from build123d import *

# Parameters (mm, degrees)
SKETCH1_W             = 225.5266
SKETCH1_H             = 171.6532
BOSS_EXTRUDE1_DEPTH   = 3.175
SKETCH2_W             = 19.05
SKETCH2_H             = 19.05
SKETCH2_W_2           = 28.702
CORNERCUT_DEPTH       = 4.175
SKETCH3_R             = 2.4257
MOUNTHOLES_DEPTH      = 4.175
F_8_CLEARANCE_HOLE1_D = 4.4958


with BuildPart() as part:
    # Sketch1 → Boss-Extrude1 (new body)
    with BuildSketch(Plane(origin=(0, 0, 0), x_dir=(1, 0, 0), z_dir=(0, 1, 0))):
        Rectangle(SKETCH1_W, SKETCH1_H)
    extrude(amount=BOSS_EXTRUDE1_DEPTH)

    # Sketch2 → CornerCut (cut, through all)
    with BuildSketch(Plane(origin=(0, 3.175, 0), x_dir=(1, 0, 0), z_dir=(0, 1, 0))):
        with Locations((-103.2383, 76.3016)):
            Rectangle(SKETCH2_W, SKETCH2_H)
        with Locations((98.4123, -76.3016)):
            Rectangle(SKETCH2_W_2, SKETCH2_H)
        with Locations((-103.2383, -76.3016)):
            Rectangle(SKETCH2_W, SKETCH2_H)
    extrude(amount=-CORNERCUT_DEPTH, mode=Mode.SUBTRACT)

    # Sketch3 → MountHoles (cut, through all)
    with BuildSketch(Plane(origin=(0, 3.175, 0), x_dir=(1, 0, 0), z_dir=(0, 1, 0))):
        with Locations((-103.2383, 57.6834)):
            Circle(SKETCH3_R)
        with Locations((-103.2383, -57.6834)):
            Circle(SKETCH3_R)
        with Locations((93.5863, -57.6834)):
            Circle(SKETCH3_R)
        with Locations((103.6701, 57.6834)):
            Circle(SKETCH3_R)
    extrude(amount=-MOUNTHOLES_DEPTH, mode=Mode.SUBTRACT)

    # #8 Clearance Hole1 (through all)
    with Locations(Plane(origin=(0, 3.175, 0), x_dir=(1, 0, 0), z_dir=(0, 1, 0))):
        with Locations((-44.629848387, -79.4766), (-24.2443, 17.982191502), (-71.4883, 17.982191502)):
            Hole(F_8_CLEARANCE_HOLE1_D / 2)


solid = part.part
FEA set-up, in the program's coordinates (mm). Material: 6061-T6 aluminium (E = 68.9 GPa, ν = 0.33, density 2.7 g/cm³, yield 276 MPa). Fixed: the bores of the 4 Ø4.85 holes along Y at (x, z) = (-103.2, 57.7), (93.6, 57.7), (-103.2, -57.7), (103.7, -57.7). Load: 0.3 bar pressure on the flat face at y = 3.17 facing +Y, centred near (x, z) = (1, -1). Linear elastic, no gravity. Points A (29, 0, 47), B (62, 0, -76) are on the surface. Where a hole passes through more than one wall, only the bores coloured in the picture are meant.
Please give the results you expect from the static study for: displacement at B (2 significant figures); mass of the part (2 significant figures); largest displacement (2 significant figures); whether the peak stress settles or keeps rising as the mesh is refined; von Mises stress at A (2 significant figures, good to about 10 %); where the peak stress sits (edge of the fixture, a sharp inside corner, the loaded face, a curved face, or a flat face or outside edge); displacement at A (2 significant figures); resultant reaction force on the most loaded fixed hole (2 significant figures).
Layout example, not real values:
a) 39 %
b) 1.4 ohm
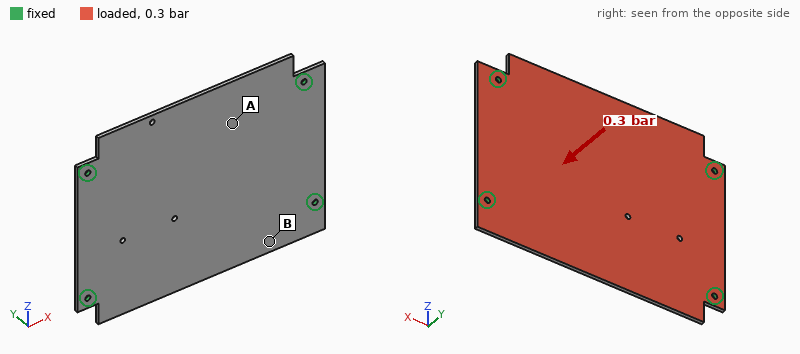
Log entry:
a) 0.49 mm
b) 320 g
c) 1.2 mm
d) keeps rising
e) 28 MPa
f) edge of the fixture
g) 0.83 mm
h) 300 N
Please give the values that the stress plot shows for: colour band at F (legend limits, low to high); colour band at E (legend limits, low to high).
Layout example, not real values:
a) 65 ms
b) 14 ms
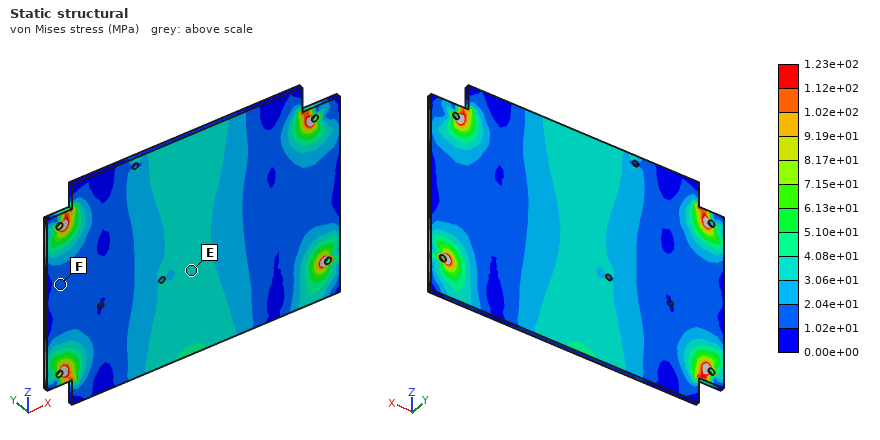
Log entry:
a) 1.02e+01 to 2.04e+01 MPa
b) 3.06e+01 to 4.08e+01 MPa
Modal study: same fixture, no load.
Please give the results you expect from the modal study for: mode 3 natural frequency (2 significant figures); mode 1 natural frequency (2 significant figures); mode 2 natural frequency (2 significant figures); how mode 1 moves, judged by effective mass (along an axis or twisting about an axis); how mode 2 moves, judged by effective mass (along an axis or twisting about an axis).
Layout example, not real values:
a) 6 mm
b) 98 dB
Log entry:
a) 780 Hz
b) 330 Hz
c) 450 Hz
d) along Y
e) twisting about X
